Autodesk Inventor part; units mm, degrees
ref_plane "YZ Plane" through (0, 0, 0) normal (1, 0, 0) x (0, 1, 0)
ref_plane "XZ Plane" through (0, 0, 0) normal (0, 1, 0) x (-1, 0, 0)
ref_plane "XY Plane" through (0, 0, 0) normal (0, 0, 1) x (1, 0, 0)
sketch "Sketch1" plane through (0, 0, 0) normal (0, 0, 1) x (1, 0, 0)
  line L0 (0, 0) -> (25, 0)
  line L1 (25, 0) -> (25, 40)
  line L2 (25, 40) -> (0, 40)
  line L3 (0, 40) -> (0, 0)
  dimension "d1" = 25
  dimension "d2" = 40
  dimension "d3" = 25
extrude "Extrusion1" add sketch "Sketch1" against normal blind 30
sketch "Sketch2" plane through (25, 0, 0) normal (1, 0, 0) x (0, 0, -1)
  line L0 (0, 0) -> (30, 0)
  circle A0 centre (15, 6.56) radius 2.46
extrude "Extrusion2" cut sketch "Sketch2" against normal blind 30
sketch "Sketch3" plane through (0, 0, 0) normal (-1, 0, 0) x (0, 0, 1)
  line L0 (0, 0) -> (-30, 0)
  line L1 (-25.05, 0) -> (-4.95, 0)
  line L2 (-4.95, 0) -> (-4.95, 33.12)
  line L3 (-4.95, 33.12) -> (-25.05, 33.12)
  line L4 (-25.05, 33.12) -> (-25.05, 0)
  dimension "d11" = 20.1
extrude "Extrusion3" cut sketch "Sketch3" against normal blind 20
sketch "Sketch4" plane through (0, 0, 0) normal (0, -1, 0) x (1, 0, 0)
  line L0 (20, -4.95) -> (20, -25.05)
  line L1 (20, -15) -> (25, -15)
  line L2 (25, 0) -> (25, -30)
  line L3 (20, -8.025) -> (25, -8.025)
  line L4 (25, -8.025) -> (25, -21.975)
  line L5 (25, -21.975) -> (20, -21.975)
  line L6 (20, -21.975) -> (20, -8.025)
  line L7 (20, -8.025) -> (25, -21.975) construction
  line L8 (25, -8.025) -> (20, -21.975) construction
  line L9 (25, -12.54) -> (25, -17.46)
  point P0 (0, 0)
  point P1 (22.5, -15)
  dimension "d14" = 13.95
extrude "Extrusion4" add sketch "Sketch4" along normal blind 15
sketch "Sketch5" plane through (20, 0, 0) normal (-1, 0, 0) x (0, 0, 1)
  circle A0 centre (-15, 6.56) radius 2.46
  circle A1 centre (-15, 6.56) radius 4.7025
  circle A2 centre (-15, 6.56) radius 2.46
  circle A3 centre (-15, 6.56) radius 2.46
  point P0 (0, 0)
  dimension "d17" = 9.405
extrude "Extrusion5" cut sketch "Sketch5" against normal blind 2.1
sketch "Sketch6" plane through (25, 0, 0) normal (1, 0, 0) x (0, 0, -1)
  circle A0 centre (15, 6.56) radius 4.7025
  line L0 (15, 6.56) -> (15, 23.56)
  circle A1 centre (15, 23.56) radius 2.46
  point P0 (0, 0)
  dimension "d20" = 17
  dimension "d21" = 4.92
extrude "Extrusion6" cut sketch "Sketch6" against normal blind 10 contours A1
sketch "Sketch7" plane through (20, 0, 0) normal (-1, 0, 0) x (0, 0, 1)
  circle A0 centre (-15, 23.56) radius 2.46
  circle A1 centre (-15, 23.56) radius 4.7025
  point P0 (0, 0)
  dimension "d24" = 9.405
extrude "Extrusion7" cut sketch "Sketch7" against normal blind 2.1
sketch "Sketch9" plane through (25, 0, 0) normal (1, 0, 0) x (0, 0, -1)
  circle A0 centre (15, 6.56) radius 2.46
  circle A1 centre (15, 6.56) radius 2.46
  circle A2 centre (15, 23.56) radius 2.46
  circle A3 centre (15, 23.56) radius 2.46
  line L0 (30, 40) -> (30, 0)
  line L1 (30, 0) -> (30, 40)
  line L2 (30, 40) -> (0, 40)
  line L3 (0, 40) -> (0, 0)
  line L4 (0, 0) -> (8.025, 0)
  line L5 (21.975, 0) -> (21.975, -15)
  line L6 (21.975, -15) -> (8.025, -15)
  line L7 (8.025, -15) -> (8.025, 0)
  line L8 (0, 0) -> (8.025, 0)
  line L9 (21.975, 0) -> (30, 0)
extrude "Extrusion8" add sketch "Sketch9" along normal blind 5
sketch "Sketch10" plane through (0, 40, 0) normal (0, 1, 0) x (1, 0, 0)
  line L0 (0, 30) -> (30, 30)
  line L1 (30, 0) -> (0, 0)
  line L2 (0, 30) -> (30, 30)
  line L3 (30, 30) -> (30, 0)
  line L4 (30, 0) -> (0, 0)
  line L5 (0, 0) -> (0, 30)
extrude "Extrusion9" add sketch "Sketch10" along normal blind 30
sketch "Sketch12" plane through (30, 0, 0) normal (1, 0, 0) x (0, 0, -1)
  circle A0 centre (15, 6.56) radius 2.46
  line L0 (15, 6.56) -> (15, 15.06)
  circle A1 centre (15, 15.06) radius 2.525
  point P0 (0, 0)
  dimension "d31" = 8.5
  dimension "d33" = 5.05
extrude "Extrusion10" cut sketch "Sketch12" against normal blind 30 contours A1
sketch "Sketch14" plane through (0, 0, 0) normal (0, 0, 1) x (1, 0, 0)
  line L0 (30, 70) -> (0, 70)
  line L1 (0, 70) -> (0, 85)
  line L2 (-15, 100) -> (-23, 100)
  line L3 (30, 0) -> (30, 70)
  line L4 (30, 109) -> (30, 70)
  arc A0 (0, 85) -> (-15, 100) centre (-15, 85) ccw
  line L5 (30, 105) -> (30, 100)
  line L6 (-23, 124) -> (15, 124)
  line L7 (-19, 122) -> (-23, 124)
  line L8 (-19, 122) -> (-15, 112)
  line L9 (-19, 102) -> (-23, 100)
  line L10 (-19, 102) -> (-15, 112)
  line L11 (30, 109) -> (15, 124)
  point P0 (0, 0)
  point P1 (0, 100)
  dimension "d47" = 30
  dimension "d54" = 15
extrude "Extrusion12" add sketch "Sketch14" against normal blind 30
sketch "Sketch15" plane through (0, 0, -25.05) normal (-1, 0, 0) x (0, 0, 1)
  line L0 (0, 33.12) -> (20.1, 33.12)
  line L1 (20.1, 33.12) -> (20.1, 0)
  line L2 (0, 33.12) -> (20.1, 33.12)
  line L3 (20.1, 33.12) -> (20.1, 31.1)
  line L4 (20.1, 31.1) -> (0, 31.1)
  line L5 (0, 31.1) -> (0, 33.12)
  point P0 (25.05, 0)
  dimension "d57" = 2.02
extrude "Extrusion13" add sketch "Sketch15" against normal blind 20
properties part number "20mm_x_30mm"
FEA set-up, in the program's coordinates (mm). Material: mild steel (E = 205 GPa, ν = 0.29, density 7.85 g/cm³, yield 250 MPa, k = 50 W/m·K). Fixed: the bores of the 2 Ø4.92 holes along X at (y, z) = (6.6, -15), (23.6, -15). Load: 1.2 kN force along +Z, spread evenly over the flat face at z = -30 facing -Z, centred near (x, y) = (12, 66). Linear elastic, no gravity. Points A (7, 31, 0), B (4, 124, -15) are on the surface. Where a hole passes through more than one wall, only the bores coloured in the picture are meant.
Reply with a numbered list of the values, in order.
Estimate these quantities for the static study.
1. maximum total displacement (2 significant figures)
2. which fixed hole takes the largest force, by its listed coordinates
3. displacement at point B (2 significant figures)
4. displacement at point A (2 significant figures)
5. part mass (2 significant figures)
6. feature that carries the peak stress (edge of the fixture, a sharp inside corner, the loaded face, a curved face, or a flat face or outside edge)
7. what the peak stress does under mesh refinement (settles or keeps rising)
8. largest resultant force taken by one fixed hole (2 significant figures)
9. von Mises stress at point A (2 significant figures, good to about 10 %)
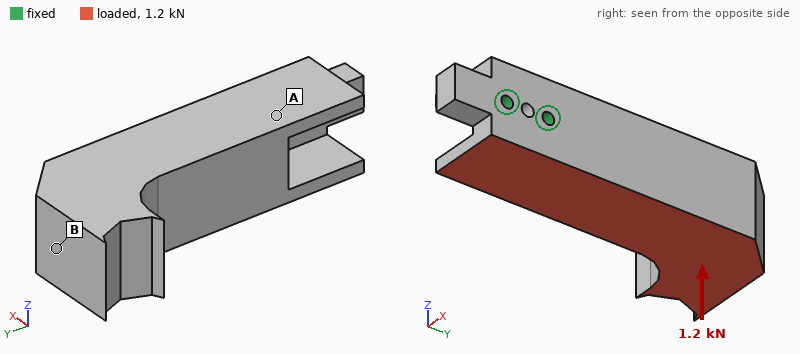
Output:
1. 43 µm
2. (23.6, -15)
3. 37 µm
4. 7.0 µm
5. 870 g
6. edge of the fixture
7. keeps rising
8. 3.3 kN
9. 12 MPa
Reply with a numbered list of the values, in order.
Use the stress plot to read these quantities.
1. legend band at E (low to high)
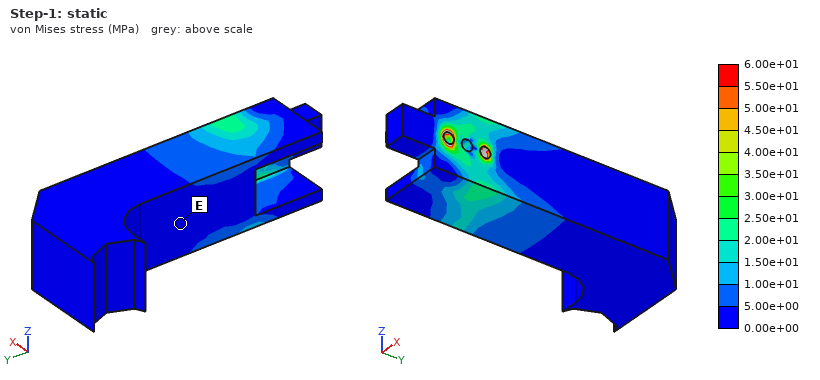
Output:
1. 0.00e+00 to 5.00e+00 MPa
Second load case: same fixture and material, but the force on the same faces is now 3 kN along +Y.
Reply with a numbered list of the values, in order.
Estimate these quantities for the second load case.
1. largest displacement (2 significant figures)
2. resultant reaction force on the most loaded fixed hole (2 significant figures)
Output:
1. 47 µm
2. 3.1 kN
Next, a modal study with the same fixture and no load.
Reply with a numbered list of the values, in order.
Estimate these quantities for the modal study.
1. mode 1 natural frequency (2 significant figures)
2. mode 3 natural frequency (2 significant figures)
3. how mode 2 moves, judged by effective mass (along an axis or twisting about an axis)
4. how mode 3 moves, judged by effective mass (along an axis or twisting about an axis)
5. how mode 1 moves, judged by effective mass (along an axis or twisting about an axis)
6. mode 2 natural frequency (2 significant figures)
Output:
1. 930 Hz
2. 2900 Hz
3. along Z
4. twisting about Y
5. along X
6. 1100 Hz
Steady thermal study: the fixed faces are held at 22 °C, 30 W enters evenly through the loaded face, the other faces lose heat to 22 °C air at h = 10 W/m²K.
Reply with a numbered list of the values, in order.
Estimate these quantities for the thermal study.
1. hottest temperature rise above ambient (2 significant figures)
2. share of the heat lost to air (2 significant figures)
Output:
1. 40 K
2. 14 %
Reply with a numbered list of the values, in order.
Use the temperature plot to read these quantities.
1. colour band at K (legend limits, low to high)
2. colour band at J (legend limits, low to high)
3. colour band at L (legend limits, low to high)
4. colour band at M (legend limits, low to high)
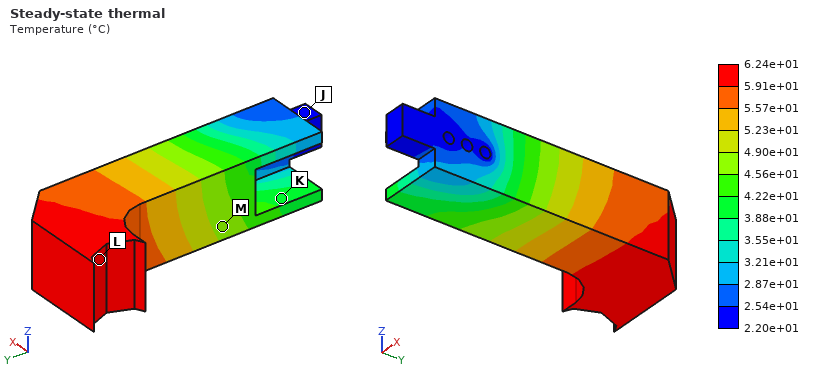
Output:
1. 3.88e+01 to 4.22e+01 °C
2. 2.20e+01 to 2.54e+01 °C
3. 5.91e+01 to 6.24e+01 °C
4. 4.56e+01 to 4.90e+01 °C
